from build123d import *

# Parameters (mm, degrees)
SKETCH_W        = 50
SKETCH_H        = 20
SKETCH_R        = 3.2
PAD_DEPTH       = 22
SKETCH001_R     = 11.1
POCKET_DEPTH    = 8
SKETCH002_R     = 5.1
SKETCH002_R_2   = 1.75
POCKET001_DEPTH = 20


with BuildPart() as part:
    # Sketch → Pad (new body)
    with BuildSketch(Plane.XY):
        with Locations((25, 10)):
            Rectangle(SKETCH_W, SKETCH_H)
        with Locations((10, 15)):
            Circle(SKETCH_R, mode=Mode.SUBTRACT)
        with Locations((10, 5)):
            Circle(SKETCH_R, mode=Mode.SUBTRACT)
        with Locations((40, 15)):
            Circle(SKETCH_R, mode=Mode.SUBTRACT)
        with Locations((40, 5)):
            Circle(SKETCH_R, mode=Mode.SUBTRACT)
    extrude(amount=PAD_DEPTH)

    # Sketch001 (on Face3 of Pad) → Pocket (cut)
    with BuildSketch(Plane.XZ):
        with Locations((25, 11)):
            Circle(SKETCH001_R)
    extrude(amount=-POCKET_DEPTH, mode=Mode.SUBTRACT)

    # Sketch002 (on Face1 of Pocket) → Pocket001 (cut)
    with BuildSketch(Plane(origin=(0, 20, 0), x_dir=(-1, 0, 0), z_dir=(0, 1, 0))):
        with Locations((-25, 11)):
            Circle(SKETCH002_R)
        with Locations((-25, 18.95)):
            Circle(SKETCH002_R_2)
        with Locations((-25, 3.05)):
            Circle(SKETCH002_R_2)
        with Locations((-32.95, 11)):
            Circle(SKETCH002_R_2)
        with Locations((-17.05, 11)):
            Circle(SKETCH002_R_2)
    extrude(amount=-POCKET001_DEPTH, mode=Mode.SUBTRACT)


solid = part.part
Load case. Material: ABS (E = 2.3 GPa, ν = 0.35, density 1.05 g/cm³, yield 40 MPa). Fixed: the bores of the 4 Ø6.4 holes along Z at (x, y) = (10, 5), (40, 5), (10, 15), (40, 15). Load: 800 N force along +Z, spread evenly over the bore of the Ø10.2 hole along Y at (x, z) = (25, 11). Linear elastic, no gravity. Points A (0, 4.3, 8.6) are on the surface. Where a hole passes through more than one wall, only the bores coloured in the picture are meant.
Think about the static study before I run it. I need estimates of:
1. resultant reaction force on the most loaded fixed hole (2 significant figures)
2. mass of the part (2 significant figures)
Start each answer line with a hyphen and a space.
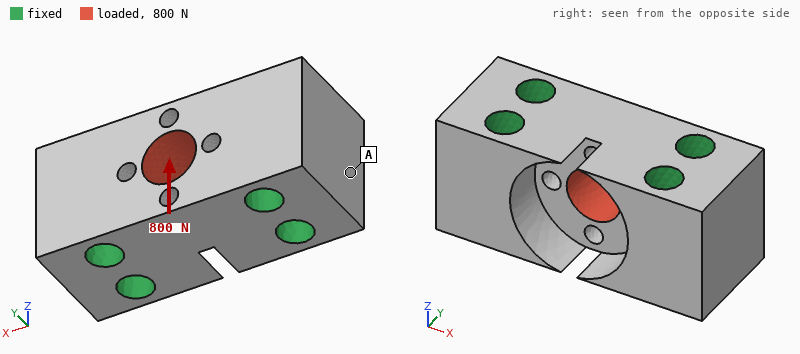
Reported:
- 310 N
- 15 g
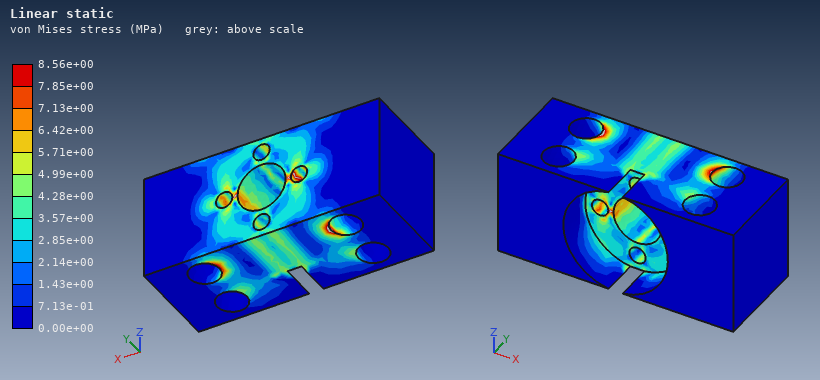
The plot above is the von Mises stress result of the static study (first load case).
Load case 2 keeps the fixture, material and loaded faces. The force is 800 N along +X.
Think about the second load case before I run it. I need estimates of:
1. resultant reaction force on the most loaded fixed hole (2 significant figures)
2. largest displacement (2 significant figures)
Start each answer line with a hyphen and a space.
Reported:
- 320 N
- 15 µm
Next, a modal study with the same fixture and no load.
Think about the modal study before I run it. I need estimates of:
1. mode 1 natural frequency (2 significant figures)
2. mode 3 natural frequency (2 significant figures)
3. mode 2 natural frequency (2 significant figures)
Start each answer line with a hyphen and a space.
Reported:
- 17 kHz
- 19 kHz
- 18 kHz
